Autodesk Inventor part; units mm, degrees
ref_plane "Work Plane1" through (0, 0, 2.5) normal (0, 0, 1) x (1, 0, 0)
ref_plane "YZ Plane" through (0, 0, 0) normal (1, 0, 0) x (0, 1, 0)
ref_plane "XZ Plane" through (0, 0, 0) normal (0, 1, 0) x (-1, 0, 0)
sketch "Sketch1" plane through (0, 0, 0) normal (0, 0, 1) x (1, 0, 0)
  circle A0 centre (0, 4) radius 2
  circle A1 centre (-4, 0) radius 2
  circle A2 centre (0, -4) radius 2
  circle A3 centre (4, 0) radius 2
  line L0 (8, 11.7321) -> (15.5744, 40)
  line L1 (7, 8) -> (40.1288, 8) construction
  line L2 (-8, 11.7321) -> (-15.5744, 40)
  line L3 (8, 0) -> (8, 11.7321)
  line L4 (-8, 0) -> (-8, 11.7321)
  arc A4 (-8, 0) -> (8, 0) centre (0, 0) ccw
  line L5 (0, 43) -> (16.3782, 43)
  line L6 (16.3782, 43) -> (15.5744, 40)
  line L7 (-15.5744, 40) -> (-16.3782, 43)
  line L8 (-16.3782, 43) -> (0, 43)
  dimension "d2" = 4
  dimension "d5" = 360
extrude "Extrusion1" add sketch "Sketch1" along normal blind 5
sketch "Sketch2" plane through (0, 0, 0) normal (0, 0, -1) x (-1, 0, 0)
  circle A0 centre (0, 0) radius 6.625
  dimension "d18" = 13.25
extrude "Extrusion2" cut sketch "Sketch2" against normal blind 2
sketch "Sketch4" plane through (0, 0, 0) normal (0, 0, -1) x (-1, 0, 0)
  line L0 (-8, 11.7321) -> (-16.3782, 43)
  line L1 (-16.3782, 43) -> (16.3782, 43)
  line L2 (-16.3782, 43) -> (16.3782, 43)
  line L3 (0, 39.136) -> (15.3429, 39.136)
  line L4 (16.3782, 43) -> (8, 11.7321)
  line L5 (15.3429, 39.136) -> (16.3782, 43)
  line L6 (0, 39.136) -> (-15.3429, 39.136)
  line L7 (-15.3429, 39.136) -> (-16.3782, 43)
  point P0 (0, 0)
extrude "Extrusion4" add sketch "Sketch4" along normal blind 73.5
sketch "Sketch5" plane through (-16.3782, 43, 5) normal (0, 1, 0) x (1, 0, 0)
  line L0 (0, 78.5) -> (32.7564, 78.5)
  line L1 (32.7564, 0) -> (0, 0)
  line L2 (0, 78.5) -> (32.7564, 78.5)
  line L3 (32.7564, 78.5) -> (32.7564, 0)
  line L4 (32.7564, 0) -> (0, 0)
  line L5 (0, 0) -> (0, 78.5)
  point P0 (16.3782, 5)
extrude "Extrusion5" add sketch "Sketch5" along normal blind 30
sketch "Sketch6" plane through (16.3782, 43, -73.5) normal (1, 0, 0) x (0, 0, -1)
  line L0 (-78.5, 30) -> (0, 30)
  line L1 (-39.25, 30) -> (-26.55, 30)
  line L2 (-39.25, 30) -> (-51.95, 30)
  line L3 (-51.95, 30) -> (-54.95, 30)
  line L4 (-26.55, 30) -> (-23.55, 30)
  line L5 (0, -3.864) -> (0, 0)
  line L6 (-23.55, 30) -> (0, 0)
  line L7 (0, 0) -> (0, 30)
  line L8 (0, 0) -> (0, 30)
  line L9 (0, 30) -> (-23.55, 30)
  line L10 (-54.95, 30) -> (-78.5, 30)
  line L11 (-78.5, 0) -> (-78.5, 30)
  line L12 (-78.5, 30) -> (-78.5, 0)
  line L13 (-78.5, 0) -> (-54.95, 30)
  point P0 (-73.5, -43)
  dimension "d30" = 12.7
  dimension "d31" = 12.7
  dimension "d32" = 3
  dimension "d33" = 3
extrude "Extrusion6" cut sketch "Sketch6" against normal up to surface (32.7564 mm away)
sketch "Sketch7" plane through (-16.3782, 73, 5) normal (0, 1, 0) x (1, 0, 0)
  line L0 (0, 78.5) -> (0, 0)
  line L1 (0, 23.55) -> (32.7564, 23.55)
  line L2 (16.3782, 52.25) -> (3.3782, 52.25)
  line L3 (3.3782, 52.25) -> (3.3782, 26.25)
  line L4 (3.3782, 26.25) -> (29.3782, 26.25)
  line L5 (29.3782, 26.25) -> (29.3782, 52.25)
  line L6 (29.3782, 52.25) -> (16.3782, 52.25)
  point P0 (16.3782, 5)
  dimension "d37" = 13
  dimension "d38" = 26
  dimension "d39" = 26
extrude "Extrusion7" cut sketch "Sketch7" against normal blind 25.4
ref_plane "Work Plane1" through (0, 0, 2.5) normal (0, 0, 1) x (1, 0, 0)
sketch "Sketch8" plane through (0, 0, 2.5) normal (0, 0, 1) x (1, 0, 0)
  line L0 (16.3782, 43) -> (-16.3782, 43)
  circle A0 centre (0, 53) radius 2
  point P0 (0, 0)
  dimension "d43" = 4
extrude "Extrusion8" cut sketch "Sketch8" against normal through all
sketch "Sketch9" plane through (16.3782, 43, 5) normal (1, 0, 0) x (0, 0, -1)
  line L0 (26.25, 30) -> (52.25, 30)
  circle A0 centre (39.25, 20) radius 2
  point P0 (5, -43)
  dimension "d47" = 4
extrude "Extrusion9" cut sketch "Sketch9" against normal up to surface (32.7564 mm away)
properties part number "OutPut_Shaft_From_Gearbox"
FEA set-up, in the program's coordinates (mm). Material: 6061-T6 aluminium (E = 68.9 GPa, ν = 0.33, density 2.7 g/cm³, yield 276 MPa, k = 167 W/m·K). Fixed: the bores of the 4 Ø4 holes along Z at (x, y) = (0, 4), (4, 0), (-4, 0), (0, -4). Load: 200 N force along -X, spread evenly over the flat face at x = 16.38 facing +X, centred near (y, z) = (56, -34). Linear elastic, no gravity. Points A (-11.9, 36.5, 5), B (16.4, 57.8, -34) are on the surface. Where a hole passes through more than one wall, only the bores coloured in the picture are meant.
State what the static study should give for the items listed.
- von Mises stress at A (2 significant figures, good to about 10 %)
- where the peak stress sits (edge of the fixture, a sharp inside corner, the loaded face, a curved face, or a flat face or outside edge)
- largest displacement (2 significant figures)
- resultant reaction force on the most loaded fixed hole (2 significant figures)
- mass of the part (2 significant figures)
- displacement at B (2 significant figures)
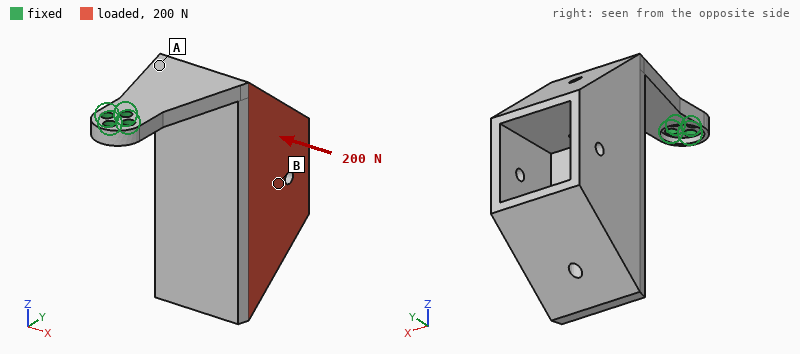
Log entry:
34 MPa
edge of the fixture
1.1 mm
830 N
140 g
0.63 mm
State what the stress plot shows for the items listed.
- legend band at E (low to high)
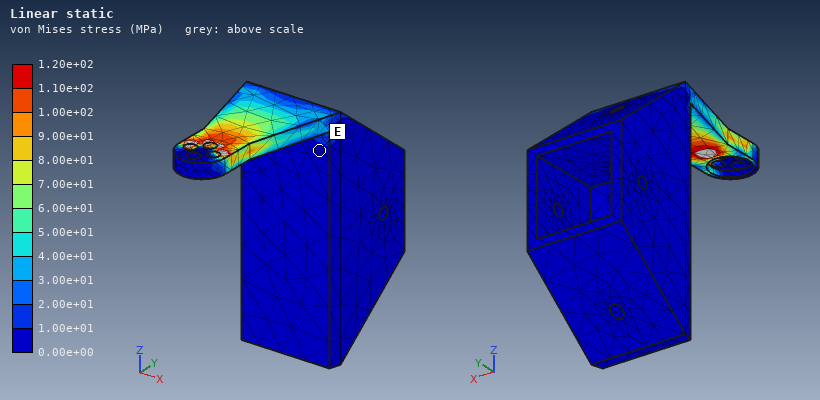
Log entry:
0.00e+00 to 1.00e+01 MPa
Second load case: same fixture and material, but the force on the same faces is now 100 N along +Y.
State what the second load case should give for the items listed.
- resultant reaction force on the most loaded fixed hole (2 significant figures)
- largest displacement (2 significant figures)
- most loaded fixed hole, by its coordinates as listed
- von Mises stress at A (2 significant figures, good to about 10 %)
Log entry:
380 N
0.84 mm
(0, 4)
29 MPa
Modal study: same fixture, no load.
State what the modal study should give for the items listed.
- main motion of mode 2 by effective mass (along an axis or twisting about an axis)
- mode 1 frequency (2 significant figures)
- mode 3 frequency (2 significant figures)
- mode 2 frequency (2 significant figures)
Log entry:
along X
160 Hz
910 Hz
230 Hz
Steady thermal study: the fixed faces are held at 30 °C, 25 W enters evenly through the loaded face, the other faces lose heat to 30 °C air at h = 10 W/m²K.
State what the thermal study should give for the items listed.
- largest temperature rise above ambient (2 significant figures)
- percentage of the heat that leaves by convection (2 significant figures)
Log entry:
55 K
25 %
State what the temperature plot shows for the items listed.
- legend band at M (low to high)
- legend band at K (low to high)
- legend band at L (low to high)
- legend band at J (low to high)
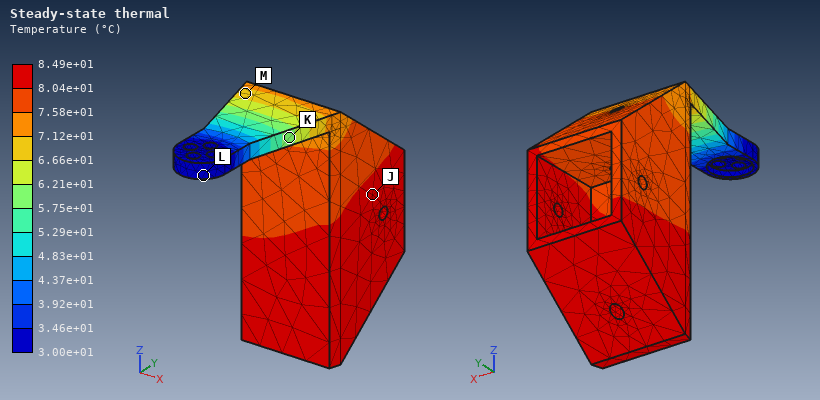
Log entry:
6.66e+01 to 7.12e+01 °C
5.75e+01 to 6.21e+01 °C
3.00e+01 to 3.46e+01 °C
8.04e+01 to 8.49e+01 °C
